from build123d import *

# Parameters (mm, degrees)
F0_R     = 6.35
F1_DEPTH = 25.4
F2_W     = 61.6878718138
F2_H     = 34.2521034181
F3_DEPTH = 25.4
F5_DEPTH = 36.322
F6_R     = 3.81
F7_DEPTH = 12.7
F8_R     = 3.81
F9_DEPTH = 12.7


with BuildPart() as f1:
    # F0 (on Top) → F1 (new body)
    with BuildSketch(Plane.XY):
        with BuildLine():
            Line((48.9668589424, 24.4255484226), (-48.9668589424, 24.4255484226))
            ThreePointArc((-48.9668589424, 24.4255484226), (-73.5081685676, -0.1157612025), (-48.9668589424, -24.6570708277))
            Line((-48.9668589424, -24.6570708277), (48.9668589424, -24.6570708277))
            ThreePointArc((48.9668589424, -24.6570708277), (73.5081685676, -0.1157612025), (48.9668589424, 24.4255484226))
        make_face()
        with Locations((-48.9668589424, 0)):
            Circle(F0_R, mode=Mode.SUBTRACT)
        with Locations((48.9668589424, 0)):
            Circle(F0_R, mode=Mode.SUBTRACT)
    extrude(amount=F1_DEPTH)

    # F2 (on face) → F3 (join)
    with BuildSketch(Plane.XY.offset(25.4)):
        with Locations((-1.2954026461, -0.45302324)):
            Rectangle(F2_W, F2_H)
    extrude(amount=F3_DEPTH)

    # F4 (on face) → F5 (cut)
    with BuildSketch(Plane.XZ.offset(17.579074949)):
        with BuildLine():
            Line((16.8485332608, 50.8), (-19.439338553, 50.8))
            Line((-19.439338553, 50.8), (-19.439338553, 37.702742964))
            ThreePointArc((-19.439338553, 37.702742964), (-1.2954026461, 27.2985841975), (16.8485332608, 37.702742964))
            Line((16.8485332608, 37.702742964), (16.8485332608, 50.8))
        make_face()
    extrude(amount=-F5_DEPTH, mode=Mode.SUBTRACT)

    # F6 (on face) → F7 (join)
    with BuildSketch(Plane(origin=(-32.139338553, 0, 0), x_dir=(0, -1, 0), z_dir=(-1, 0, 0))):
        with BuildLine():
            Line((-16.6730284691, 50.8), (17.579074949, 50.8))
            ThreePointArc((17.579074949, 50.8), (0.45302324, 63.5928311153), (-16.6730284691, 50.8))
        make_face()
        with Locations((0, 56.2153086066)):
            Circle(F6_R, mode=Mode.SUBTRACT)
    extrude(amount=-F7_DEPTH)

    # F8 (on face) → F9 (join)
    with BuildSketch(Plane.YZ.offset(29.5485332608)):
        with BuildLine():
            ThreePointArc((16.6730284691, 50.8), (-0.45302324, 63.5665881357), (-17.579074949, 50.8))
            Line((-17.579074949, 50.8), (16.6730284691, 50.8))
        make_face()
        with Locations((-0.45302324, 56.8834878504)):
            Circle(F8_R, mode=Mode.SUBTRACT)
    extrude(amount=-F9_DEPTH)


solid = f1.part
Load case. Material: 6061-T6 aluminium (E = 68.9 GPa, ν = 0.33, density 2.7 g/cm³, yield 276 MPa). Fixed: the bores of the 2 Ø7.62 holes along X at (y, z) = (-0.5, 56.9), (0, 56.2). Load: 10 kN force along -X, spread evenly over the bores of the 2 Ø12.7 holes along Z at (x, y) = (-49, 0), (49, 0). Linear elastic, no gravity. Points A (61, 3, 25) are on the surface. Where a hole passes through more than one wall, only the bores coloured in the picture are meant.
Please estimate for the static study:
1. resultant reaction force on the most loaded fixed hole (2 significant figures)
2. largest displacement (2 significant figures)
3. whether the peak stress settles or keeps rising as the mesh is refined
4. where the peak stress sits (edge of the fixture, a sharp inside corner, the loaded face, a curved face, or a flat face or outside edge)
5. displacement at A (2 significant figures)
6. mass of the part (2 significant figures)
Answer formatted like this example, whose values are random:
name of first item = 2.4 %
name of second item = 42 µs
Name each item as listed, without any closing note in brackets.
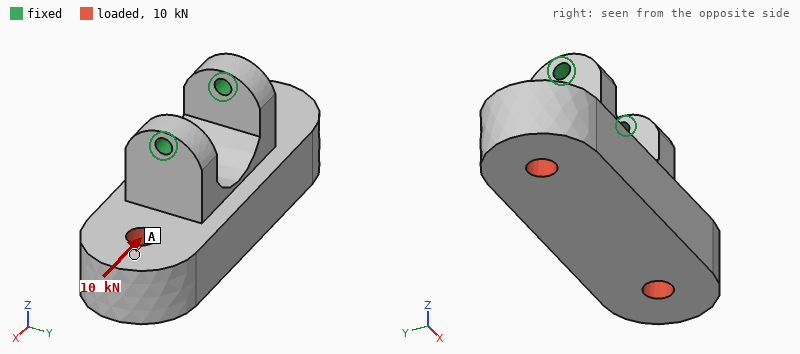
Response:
resultant reaction force on the most loaded fixed hole = 8.1 kN
largest displacement = 64 µm
whether the peak stress settles or keeps rising as the mesh is refined = keeps rising
where the peak stress sits = edge of the fixture
displacement at A = 52 µm
mass of the part = 540 g
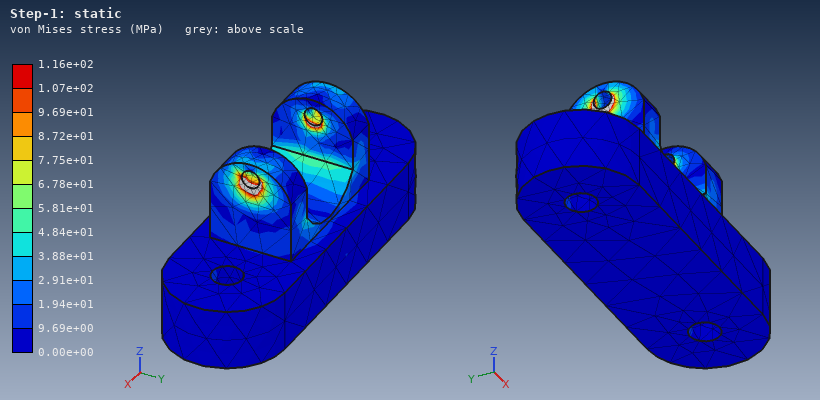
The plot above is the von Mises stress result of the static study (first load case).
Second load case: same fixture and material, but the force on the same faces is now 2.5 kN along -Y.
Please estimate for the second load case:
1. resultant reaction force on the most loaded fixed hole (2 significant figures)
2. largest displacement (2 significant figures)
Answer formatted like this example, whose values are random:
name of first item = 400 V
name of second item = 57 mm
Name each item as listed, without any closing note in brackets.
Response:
resultant reaction force on the most loaded fixed hole = 1.3 kN
largest displacement = 84 µm
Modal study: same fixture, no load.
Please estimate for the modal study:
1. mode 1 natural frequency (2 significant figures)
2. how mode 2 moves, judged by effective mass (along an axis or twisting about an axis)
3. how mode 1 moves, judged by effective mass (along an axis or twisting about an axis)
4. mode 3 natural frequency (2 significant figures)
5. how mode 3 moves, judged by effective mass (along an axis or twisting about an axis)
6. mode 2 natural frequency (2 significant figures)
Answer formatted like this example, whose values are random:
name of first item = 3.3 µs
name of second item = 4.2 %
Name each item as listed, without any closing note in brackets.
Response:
mode 1 natural frequency = 1500 Hz
how mode 2 moves, judged by effective mass = twisting about Z
how mode 1 moves, judged by effective mass = along Y
mode 3 natural frequency = 3100 Hz
how mode 3 moves, judged by effective mass = along X
mode 2 natural frequency = 2400 Hz
